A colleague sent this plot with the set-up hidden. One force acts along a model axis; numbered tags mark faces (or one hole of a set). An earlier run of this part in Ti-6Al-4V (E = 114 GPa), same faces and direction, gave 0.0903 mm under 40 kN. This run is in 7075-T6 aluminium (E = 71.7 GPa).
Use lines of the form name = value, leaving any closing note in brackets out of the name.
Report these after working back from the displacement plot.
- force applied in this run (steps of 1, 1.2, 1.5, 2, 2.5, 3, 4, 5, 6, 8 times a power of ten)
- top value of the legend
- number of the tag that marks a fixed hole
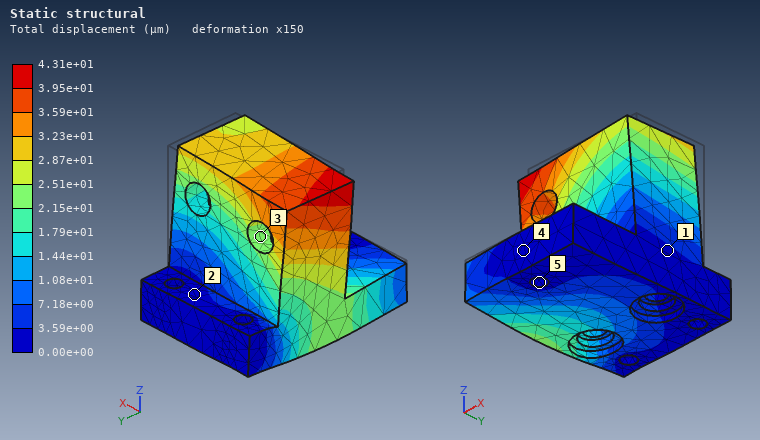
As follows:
force applied in this run = 12 kN
top value of the legend = 4.31e+01 µm
number of the tag that marks a fixed hole = 5
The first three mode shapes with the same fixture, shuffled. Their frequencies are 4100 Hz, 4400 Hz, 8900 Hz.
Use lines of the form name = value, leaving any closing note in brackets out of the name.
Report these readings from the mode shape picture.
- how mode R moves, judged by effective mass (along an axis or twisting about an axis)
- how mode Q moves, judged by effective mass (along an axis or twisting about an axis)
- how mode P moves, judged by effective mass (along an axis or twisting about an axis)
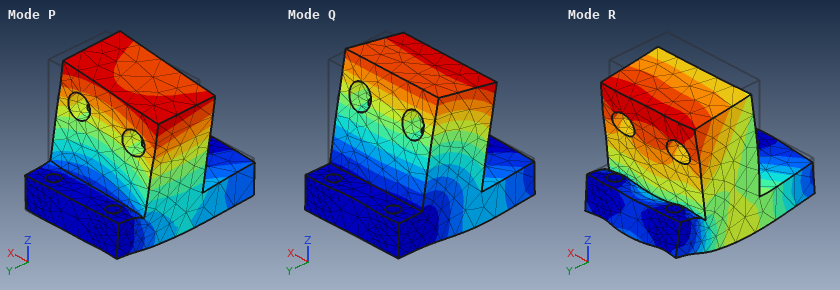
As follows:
how mode R moves, judged by effective mass = along Z
how mode Q moves, judged by effective mass = along Y
how mode P moves, judged by effective mass = along X
